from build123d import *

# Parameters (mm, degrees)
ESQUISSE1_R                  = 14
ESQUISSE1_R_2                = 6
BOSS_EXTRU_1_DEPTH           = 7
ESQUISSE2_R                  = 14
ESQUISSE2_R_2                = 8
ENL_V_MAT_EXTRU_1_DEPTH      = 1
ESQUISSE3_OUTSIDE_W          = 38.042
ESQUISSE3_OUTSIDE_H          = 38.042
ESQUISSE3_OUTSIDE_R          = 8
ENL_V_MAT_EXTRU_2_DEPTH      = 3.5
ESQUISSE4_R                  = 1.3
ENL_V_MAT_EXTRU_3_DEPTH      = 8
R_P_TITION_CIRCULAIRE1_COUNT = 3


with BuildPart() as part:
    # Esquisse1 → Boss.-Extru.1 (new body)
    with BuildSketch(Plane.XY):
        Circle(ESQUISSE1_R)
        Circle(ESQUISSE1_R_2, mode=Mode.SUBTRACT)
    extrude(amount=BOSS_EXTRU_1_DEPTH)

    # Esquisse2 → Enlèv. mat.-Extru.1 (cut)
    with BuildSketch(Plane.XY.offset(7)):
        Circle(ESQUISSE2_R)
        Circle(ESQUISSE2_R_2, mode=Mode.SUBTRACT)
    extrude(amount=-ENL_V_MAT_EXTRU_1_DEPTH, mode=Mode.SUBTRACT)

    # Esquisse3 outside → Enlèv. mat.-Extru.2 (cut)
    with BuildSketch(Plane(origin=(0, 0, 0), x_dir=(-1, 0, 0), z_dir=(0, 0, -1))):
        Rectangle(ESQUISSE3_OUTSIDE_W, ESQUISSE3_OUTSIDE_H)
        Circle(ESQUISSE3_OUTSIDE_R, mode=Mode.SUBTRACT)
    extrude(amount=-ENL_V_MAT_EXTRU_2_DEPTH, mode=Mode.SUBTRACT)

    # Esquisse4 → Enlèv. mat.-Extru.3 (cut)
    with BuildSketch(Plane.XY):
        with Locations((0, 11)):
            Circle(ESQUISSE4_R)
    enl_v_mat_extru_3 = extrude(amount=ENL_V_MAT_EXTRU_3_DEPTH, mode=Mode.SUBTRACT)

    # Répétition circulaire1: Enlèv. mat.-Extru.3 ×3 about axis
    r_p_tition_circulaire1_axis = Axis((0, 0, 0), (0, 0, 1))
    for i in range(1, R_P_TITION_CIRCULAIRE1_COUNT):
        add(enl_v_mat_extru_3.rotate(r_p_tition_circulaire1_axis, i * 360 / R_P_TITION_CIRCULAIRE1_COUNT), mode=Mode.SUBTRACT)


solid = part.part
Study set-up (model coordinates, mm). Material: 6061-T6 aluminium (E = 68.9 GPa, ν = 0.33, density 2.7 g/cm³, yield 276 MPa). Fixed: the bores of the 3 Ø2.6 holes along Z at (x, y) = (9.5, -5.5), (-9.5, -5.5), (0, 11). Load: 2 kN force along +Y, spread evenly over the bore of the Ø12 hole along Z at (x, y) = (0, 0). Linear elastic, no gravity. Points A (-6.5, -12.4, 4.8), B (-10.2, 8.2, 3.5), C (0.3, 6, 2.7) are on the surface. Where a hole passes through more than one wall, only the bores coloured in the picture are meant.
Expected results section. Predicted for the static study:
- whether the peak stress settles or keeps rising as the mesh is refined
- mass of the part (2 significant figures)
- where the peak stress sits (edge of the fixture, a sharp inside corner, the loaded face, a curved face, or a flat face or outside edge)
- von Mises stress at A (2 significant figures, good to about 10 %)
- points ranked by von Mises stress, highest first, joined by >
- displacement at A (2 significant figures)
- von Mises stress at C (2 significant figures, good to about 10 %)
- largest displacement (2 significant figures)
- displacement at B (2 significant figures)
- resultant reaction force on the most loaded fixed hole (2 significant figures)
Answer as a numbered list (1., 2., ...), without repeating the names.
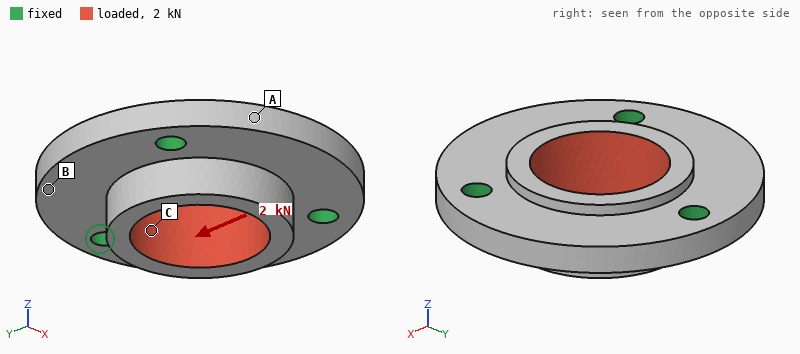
1. keeps rising
2. 4.4 g
3. edge of the fixture
4. 20 MPa
5. C > A > B
6. 5.0 µm
7. 36 MPa
8. 12 µm
9. 4.4 µm
10. 730 N
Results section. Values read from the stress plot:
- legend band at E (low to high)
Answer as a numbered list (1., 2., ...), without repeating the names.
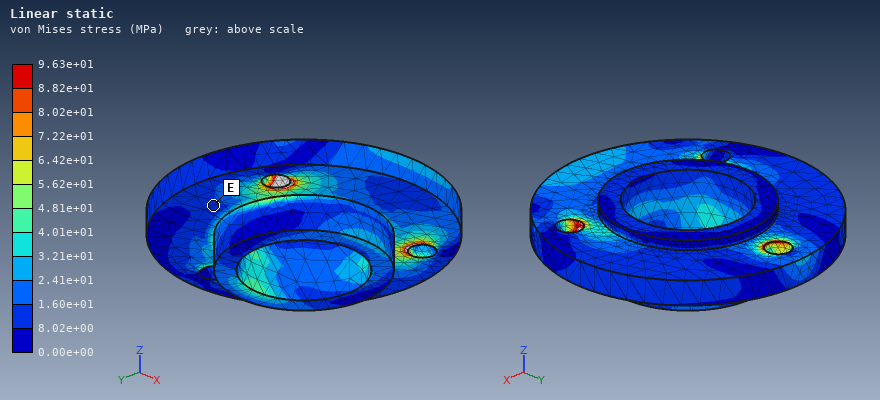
1. 8.02e+00 to 1.60e+01 MPa
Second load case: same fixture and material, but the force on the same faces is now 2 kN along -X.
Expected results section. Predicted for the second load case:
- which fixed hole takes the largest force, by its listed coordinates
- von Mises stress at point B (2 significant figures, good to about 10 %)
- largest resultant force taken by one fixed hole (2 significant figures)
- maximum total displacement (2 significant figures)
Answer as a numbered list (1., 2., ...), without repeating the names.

1. (0, 11)
2. 13 MPa
3. 770 N
4. 11 µm
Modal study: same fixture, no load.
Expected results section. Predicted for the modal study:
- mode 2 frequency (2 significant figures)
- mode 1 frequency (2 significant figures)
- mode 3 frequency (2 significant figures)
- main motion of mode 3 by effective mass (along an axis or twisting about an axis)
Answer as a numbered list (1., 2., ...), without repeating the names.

1. 24 kHz
2. 24 kHz
3. 30 kHz
4. along Z
